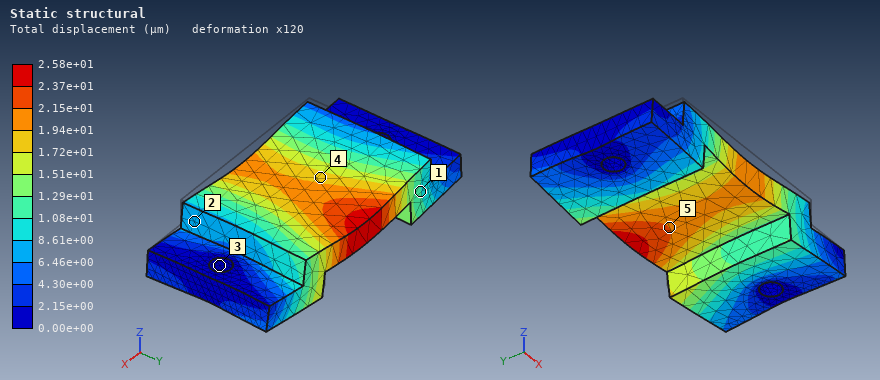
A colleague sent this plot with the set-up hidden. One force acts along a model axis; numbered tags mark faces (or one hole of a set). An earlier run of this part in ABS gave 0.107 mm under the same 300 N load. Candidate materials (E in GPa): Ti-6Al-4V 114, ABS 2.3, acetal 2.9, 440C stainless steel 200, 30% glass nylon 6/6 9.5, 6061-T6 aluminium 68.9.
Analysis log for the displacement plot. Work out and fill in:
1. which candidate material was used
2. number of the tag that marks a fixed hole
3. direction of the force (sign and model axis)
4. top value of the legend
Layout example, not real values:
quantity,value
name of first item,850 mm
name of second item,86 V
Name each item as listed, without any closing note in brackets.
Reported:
quantity,value
which candidate material was used,30% glass nylon 6/6
number of the tag that marks a fixed hole,3
direction of the force,-Z
top value of the legend,2.58e+01 µm
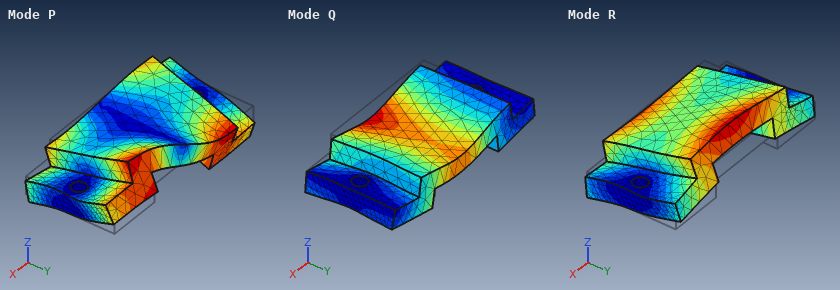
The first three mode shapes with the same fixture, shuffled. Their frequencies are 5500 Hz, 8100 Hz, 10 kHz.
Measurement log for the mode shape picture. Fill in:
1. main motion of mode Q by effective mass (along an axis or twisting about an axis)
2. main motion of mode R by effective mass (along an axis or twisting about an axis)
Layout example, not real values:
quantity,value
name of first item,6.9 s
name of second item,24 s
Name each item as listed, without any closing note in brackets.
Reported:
quantity,value
main motion of mode Q by effective mass,along Z
main motion of mode R by effective mass,along Y
